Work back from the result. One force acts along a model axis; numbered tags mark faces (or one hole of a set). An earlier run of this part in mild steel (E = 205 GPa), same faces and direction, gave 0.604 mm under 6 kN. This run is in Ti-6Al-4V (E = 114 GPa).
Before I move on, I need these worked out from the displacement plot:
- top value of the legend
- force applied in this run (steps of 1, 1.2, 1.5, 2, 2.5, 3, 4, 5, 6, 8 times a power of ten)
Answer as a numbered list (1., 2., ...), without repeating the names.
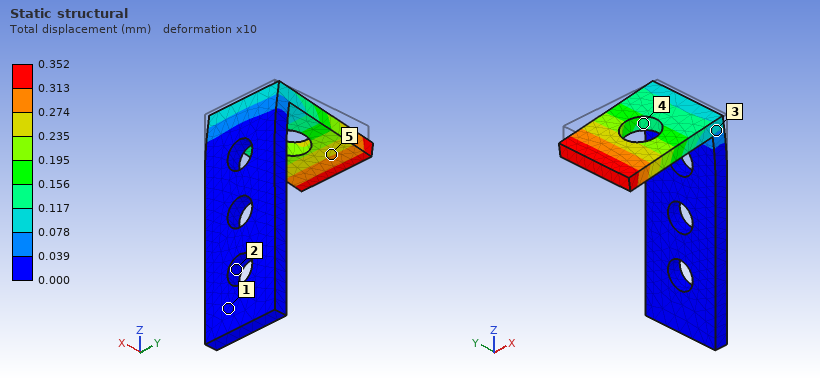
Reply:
1. 0.352 mm
2. 2 kN
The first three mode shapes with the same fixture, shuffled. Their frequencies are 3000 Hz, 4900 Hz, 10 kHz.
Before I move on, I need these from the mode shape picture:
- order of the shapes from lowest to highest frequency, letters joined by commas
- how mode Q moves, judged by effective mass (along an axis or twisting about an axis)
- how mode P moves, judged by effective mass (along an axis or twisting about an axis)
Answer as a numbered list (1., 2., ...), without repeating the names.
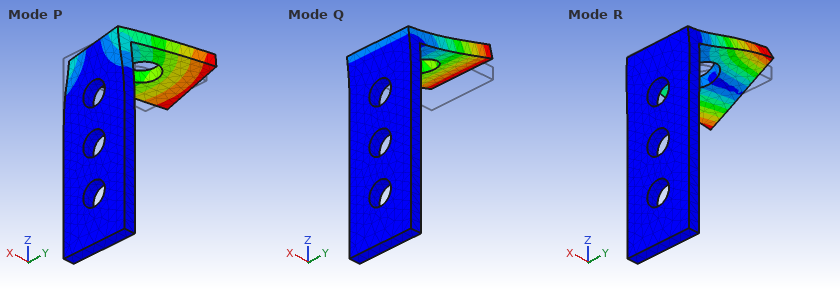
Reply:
1. Q, P, R
2. along Z
3. along Y
